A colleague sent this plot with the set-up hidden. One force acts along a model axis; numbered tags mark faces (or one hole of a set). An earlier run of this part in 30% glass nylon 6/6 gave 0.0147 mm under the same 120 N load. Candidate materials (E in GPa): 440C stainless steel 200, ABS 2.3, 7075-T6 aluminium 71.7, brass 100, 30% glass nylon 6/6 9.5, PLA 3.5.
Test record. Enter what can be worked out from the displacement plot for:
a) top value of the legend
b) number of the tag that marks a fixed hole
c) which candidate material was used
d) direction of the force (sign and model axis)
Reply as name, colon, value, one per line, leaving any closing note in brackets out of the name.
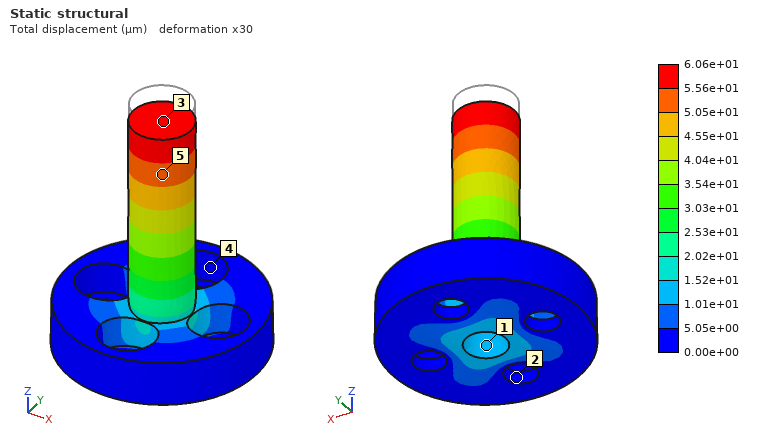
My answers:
top value of the legend: 6.06e+01 µm
number of the tag that marks a fixed hole: 2
which candidate material was used: ABS
direction of the force: -Z
